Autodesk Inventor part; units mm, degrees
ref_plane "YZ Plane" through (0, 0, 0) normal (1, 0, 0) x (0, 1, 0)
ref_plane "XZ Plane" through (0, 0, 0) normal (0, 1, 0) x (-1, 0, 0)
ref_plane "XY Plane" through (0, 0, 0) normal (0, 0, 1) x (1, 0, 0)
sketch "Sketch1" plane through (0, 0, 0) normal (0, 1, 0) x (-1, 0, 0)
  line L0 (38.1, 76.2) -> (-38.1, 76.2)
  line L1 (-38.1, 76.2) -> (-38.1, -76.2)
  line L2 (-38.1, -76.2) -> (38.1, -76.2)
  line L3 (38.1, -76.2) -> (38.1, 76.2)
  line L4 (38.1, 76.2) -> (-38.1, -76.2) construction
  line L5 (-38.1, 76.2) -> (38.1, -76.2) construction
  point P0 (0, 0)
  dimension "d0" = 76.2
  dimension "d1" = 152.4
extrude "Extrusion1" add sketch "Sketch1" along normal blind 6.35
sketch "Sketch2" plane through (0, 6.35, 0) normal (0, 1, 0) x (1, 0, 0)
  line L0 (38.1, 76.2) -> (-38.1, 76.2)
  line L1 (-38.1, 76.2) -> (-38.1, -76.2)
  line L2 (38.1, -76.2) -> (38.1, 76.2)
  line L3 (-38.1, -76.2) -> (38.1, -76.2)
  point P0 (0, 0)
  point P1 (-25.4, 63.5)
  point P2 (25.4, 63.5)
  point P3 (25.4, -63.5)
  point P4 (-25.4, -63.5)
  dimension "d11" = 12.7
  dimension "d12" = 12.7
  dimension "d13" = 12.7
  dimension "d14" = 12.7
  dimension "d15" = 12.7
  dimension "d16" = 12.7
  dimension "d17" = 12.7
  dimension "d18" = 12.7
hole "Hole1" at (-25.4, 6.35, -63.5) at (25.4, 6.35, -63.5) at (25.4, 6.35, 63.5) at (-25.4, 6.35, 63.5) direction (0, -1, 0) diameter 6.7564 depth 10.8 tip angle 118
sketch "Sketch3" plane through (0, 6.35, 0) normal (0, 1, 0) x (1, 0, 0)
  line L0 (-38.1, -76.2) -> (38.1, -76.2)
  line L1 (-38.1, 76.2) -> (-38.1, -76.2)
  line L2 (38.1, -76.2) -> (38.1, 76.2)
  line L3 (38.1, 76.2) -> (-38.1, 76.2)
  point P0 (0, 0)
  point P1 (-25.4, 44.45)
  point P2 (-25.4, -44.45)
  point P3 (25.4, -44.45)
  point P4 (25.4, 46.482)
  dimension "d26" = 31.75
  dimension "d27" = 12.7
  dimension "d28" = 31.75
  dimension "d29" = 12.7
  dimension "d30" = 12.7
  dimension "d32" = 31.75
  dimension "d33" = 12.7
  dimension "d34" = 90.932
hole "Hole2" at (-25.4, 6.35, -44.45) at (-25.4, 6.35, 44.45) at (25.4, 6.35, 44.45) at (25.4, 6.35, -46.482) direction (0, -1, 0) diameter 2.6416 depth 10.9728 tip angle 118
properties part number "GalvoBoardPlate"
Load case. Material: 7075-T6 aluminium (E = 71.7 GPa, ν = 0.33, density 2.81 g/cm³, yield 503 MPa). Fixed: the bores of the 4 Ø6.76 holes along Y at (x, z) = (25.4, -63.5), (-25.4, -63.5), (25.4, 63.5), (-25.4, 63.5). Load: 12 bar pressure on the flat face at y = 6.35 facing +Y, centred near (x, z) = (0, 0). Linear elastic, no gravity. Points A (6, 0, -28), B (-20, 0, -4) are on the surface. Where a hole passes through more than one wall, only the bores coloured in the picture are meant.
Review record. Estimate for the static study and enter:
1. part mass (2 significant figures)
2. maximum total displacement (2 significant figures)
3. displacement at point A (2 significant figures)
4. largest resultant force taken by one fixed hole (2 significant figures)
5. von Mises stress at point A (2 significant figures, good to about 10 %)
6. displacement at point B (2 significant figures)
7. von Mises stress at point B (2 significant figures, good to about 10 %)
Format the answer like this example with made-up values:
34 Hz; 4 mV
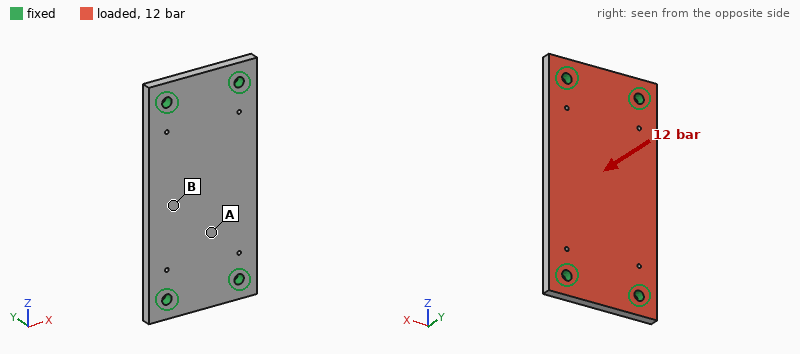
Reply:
200 g; 0.59 mm; 0.38 mm; 3.4 kN; 47 MPa; 0.55 mm; 110 MPa
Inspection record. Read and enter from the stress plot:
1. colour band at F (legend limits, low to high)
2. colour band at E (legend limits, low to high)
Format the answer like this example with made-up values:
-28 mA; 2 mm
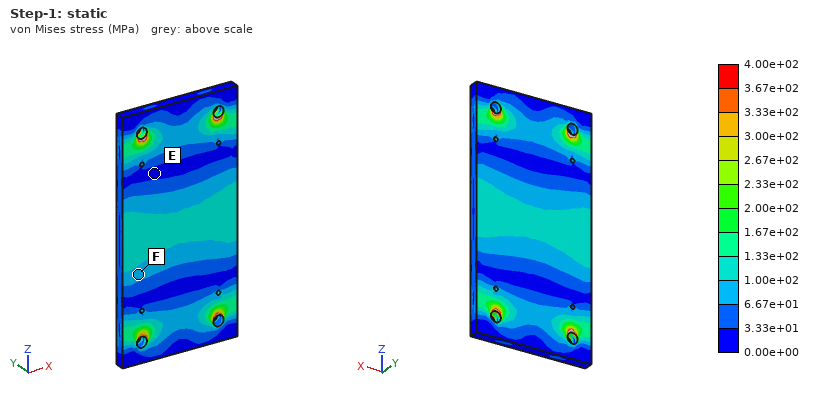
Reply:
6.67e+01 to 1.00e+02 MPa; 0.00e+00 to 3.33e+01 MPa
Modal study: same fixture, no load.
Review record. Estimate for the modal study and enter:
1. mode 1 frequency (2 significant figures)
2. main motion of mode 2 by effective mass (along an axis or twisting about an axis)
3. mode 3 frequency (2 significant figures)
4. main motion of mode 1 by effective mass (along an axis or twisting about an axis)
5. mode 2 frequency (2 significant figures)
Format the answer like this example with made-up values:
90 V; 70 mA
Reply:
2000 Hz; twisting about Z; 5300 Hz; along Y; 3000 Hz
